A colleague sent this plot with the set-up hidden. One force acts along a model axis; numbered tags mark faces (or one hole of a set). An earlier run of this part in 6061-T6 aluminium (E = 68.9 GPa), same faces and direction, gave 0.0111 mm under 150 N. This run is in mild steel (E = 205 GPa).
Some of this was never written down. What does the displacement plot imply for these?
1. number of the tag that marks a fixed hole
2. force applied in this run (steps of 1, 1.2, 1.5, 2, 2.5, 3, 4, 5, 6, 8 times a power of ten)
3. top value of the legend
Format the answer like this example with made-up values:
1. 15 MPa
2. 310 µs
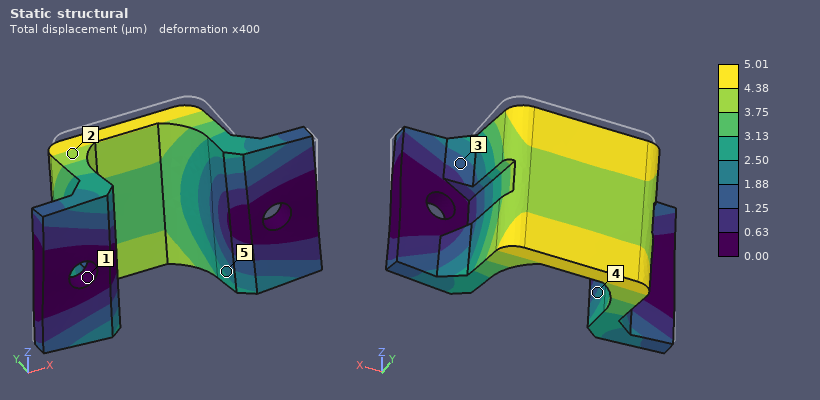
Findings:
1. 1
2. 200 N
3. 5.01 µm
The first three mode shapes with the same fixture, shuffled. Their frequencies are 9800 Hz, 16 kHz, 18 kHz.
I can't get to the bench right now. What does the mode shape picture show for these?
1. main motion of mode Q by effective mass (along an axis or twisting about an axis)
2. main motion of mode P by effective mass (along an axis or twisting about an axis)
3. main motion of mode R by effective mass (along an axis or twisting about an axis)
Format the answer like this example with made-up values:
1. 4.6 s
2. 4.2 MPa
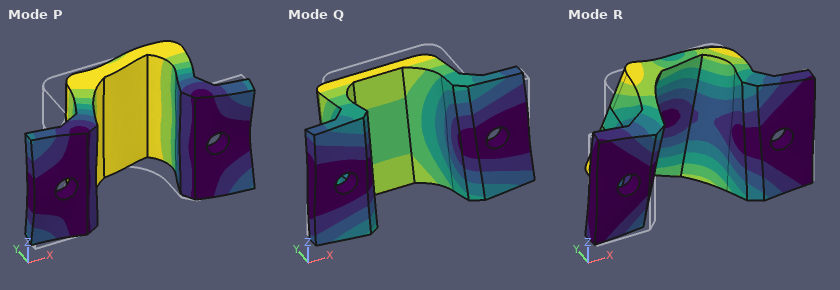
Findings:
1. along Z
2. along X
3. twisting about Y
